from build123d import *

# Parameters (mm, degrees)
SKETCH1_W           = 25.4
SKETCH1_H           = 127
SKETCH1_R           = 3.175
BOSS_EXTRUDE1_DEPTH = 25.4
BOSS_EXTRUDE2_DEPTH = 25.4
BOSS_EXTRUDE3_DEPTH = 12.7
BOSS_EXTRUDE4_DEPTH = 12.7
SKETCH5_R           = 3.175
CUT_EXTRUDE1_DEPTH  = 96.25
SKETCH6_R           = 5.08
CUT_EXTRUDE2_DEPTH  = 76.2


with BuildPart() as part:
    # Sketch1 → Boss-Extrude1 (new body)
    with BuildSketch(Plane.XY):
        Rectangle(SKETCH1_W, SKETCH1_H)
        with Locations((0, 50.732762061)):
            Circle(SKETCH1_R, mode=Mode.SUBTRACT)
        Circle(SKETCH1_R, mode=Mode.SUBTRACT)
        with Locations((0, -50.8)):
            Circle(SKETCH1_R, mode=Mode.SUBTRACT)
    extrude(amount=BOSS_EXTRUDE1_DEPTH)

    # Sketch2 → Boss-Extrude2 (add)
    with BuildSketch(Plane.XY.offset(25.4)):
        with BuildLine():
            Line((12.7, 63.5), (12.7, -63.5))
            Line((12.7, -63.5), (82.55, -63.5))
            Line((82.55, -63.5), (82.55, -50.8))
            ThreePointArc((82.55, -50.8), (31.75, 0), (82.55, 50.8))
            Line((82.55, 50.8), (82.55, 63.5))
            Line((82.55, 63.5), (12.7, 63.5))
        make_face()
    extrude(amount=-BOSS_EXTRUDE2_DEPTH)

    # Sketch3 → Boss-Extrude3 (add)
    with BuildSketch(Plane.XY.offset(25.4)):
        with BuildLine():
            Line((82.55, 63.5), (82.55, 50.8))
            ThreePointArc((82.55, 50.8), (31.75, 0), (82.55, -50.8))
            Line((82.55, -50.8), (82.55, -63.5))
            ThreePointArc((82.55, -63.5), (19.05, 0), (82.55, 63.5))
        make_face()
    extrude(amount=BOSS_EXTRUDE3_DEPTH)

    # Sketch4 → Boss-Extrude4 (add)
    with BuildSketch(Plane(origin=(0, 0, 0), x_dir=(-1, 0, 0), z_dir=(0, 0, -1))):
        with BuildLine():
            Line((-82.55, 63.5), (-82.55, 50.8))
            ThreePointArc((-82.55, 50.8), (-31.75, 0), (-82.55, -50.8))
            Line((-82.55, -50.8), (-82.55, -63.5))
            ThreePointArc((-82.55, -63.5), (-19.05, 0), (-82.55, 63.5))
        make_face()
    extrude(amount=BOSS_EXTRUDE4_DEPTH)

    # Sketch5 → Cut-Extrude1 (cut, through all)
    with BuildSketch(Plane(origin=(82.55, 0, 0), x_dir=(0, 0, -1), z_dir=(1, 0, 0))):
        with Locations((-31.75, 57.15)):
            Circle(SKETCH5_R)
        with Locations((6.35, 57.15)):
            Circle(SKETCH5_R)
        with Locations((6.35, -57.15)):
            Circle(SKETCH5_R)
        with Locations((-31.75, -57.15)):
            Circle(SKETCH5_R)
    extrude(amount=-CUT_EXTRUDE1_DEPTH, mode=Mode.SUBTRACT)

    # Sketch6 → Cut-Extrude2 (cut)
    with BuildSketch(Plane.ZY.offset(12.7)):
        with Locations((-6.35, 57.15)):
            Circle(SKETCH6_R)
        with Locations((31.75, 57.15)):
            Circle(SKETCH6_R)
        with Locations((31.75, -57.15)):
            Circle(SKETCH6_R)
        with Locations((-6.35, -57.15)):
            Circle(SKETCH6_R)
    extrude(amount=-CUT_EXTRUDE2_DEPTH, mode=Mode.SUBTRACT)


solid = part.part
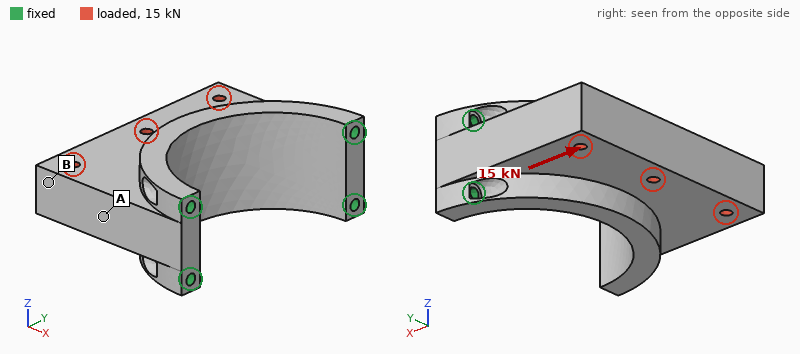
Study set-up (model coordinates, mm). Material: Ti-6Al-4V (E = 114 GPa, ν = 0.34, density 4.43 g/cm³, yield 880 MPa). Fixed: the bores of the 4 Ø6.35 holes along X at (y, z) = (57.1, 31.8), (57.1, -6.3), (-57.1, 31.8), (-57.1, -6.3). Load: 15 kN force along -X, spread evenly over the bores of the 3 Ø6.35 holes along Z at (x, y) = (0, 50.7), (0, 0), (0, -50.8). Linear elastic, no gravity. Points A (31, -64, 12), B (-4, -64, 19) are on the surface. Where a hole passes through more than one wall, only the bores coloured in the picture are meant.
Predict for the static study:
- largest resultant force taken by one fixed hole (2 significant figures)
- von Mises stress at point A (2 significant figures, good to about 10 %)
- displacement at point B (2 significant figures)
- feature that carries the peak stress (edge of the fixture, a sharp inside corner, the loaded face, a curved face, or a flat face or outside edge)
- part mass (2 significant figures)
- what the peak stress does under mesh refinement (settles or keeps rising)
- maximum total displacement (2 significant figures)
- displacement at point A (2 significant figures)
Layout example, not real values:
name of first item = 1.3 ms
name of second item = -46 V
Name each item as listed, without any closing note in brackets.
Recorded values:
largest resultant force taken by one fixed hole = 4.1 kN
von Mises stress at point A = 8.0 MPa
displacement at point B = 6.5 µm
feature that carries the peak stress = edge of the fixture
part mass = 1.1 kg
what the peak stress does under mesh refinement = keeps rising
maximum total displacement = 8.9 µm
displacement at point A = 4.7 µm
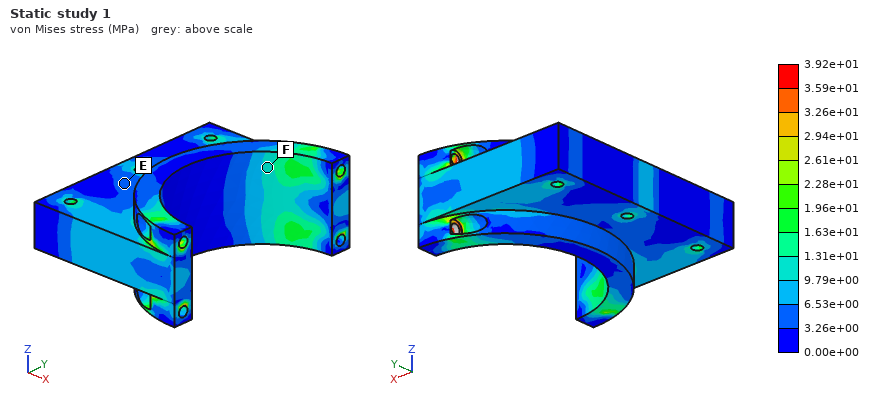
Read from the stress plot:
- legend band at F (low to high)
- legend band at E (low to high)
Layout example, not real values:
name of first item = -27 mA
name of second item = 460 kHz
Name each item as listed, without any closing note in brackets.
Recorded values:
legend band at F = 9.79e+00 to 1.31e+01 MPa
legend band at E = 3.26e+00 to 6.53e+00 MPa
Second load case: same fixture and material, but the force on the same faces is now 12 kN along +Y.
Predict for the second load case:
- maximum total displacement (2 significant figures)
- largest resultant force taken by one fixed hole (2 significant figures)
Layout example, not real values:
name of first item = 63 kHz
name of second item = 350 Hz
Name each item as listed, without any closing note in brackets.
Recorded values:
maximum total displacement = 25 µm
largest resultant force taken by one fixed hole = 4.7 kN
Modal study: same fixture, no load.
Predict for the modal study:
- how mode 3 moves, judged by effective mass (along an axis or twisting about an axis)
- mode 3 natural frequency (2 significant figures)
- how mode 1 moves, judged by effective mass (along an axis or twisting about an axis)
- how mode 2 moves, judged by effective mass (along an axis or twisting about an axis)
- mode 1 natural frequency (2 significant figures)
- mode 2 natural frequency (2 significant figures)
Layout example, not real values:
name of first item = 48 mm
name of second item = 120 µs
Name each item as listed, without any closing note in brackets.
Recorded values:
how mode 3 moves, judged by effective mass = twisting about X
mode 3 natural frequency = 4600 Hz
how mode 1 moves, judged by effective mass = along Z
how mode 2 moves, judged by effective mass = along Y
mode 1 natural frequency = 2600 Hz
mode 2 natural frequency = 4100 Hz
